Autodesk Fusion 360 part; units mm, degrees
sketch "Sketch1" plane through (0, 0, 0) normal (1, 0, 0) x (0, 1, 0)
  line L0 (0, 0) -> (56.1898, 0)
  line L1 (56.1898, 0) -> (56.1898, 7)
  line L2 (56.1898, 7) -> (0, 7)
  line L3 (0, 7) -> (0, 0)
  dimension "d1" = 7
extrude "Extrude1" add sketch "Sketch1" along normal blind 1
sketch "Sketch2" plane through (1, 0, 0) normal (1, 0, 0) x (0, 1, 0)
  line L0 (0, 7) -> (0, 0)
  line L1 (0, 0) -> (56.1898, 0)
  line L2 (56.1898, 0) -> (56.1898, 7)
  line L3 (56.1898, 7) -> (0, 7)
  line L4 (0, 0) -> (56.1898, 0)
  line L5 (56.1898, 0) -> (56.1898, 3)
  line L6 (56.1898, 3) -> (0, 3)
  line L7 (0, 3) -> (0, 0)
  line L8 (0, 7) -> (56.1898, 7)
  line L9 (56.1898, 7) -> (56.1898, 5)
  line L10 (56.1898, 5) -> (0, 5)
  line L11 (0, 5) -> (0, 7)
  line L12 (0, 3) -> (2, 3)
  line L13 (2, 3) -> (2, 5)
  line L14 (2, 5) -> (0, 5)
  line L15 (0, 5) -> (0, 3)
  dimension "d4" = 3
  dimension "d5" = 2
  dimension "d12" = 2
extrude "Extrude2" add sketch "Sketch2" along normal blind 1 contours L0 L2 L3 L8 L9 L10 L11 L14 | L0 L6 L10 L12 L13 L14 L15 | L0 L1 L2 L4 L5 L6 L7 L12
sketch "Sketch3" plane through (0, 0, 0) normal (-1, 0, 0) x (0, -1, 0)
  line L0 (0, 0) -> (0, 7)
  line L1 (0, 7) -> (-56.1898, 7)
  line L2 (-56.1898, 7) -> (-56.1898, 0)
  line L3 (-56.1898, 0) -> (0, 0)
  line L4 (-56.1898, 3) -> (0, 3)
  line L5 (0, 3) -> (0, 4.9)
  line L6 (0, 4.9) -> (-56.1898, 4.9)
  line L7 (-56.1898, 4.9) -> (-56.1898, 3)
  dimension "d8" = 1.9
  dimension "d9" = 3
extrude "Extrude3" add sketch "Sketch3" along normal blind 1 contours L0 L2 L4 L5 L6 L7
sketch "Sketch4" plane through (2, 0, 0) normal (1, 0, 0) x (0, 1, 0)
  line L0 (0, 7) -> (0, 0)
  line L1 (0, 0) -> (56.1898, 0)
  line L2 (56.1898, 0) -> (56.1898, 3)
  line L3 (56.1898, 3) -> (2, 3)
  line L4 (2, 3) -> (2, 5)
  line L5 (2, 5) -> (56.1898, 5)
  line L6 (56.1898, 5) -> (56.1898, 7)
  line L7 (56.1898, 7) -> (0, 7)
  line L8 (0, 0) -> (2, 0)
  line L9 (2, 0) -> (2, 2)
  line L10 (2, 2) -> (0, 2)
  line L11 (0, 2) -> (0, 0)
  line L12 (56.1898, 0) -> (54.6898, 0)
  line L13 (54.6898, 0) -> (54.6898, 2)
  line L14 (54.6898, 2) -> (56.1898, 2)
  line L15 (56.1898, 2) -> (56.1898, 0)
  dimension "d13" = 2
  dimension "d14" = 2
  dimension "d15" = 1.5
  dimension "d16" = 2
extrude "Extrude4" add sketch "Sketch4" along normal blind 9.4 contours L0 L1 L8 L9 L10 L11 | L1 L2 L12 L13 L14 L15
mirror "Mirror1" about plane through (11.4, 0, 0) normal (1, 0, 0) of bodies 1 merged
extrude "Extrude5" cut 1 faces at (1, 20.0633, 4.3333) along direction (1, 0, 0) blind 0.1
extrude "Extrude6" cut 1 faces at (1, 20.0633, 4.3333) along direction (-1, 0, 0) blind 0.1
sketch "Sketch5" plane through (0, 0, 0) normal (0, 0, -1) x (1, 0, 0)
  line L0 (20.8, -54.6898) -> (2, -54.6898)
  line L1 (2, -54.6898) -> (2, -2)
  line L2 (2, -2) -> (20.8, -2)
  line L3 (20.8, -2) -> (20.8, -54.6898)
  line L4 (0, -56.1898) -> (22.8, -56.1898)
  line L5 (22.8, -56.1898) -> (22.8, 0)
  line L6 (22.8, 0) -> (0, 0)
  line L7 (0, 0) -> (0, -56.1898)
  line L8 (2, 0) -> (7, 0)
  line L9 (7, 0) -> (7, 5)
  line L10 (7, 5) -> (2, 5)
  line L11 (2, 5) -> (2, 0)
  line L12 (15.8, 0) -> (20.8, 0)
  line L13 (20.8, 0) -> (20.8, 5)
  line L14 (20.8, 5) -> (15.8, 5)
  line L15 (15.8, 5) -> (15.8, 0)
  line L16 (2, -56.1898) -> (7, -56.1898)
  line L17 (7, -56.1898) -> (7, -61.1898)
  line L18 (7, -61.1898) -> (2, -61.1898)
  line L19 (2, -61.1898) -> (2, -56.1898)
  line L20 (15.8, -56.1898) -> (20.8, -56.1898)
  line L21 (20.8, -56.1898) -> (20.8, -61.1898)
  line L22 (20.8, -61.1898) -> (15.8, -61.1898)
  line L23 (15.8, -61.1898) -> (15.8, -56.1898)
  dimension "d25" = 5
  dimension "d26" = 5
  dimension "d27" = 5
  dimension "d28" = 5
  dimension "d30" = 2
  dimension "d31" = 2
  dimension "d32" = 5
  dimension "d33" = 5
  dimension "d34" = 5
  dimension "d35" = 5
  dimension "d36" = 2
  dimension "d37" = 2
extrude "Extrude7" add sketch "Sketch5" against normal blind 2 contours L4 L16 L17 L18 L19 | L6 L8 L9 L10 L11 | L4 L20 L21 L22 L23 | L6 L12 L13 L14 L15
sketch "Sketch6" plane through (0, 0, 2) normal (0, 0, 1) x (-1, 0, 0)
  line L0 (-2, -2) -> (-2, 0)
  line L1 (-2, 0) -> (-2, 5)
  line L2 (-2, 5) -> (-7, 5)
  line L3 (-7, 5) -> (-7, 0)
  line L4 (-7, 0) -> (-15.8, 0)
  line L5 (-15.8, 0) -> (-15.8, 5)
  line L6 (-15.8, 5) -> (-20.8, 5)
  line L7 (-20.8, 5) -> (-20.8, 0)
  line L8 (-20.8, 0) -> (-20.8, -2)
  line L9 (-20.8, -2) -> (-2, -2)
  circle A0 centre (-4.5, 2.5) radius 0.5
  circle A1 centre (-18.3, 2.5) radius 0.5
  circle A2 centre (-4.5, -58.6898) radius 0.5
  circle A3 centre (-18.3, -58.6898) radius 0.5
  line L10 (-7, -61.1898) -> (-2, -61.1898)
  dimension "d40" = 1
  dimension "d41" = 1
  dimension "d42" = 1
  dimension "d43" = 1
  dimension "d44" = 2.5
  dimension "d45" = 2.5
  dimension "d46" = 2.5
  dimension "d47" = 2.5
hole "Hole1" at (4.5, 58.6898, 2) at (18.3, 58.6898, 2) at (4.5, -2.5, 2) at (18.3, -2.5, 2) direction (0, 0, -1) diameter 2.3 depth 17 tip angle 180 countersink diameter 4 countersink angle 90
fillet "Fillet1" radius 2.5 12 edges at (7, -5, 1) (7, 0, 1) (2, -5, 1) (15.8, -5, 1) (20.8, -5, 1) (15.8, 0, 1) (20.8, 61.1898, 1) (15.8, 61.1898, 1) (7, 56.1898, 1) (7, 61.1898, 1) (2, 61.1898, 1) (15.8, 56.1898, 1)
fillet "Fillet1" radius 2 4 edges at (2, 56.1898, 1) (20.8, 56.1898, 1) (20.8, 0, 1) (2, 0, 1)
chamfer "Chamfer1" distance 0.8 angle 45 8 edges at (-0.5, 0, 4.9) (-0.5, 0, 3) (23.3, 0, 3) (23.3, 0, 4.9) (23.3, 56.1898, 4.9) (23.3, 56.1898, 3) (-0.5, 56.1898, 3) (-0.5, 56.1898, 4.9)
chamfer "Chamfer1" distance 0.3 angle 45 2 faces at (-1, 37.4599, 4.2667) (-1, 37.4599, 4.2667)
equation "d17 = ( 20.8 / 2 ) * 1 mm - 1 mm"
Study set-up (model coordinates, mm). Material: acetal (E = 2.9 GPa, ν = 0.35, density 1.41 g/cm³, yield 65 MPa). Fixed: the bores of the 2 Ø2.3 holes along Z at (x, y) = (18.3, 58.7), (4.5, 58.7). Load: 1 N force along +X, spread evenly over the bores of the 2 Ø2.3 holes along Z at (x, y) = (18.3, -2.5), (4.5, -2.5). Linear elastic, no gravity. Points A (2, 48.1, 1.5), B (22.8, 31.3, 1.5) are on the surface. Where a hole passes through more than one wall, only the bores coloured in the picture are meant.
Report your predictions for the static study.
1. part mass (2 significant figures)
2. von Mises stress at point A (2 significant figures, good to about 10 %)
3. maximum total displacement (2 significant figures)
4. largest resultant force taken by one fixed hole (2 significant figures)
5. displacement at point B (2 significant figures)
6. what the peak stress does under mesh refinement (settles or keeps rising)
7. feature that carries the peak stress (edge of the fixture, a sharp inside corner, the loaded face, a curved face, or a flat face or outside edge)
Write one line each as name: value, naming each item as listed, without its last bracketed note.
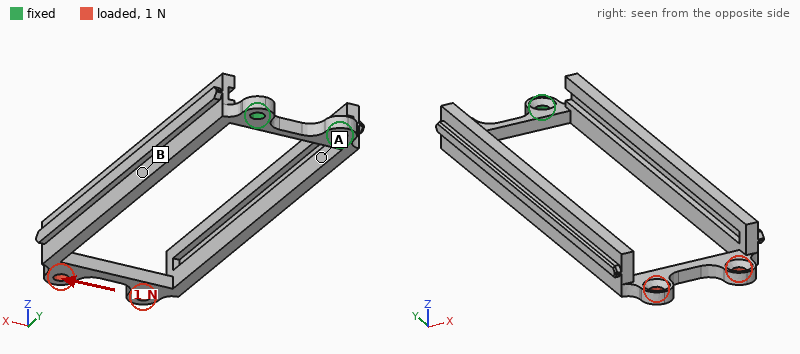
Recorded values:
part mass: 2.6 g
von Mises stress at point A: 1.6 MPa
maximum total displacement: 0.82 mm
largest resultant force taken by one fixed hole: 2.0 N
displacement at point B: 0.36 mm
what the peak stress does under mesh refinement: keeps rising
feature that carries the peak stress: a sharp inside corner
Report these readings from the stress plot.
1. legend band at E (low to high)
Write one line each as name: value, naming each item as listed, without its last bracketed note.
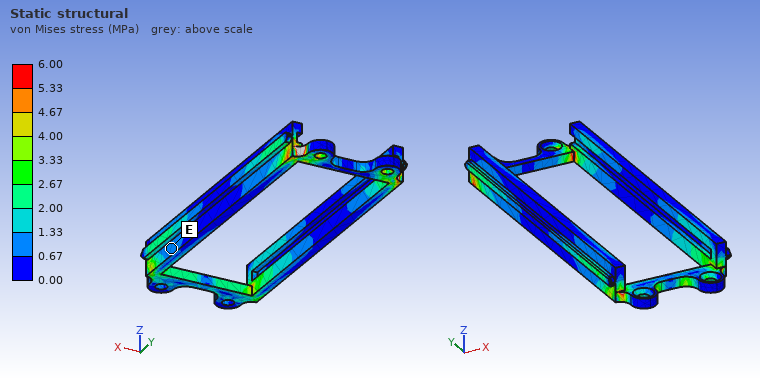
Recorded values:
legend band at E: 0.67 to 1.33 MPa
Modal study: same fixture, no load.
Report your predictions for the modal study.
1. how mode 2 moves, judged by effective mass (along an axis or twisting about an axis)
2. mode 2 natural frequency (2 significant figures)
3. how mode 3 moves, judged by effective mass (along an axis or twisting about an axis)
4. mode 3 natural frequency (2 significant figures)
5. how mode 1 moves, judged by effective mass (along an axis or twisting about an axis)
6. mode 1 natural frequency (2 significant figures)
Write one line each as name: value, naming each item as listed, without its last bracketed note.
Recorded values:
how mode 2 moves, judged by effective mass: along X
mode 2 natural frequency: 170 Hz
how mode 3 moves, judged by effective mass: twisting about Y
mode 3 natural frequency: 320 Hz
how mode 1 moves, judged by effective mass: along Z
mode 1 natural frequency: 130 Hz
